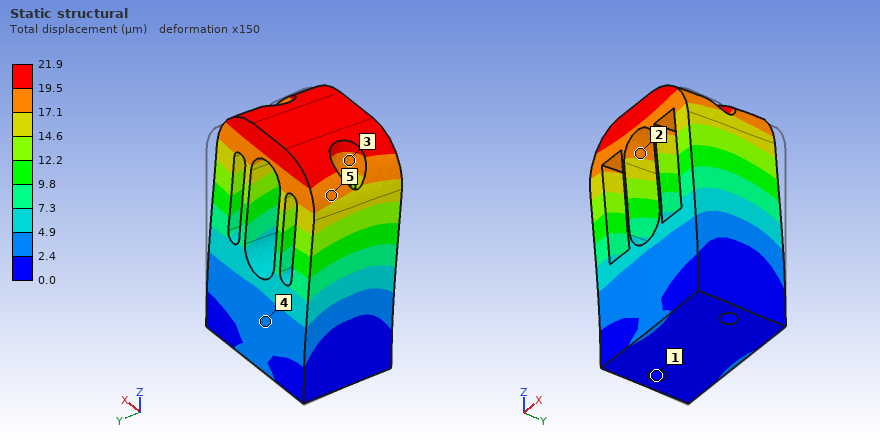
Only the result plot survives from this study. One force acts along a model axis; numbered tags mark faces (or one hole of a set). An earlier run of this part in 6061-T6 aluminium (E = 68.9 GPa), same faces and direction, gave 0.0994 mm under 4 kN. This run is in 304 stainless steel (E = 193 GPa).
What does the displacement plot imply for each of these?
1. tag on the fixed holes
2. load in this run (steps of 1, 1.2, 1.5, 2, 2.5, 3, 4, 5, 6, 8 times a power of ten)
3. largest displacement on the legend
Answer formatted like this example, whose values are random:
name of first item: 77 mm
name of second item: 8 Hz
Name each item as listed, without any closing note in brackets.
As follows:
tag on the fixed holes: 1
load in this run: 2.5 kN
largest displacement on the legend: 21.9 µm
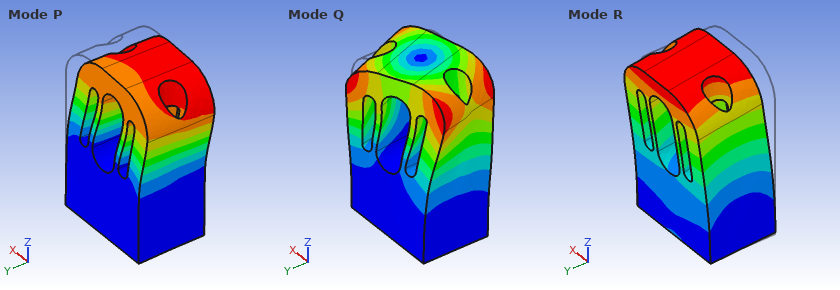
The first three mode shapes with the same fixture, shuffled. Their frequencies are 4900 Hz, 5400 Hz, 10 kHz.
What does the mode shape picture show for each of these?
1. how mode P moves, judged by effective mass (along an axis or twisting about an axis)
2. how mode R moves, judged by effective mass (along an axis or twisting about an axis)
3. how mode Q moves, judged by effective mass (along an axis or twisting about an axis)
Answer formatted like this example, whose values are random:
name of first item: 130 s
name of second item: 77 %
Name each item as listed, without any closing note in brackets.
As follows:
how mode P moves, judged by effective mass: along X
how mode R moves, judged by effective mass: along Y
how mode Q moves, judged by effective mass: twisting about Z
